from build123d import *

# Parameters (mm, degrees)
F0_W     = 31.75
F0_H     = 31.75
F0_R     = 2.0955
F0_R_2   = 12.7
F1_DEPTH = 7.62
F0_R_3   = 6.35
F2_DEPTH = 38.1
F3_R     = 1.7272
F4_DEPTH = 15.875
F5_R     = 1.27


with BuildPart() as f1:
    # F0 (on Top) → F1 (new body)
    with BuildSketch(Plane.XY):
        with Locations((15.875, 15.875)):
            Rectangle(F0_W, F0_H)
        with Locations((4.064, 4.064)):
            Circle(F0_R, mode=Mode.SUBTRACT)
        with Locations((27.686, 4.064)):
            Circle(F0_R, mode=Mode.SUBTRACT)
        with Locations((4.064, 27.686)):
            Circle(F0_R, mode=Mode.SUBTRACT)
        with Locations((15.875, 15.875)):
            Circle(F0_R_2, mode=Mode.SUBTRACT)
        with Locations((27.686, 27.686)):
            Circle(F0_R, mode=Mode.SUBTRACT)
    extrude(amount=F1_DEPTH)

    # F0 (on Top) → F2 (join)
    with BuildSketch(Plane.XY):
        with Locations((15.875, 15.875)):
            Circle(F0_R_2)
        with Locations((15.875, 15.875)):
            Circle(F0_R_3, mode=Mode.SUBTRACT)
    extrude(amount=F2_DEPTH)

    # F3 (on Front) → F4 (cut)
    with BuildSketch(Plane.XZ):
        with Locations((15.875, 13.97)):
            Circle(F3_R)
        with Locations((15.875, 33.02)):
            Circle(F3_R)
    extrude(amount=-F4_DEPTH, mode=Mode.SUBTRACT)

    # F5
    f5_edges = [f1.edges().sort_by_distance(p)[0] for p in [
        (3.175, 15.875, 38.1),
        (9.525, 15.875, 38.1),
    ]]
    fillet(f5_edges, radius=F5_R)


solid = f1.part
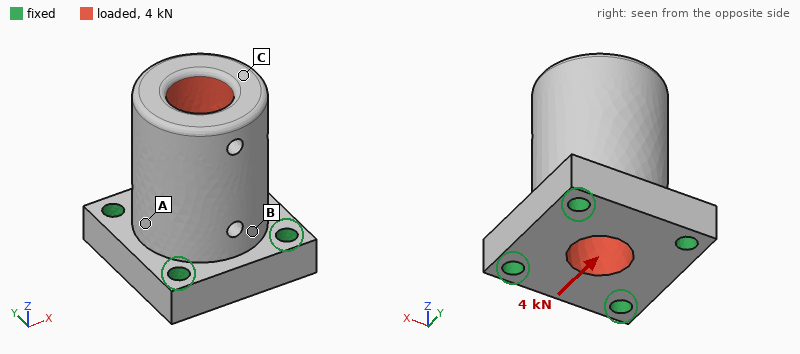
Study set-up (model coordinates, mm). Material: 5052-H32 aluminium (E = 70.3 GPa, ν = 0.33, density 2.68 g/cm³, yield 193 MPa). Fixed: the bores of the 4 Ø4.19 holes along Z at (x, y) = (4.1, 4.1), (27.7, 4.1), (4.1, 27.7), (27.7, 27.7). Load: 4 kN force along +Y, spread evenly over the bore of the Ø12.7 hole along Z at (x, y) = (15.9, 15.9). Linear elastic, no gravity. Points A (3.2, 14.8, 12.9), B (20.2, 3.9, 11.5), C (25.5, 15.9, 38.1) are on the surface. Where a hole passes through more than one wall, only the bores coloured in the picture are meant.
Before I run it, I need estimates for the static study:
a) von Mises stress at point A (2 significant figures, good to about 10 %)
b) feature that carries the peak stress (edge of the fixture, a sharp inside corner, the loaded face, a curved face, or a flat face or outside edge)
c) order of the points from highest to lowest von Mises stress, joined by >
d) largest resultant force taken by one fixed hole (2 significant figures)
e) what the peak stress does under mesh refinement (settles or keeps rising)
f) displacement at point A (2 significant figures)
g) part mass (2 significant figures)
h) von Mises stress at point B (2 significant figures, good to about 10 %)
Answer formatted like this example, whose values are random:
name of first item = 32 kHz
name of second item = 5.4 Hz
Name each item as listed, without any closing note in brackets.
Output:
von Mises stress at point A = 15 MPa
feature that carries the peak stress = edge of the fixture
order of the points from highest to lowest von Mises stress, joined by > = B > A > C
largest resultant force taken by one fixed hole = 1.7 kN
what the peak stress does under mesh refinement = keeps rising
displacement at point A = 6.6 µm
part mass = 47 g
von Mises stress at point B = 25 MPa
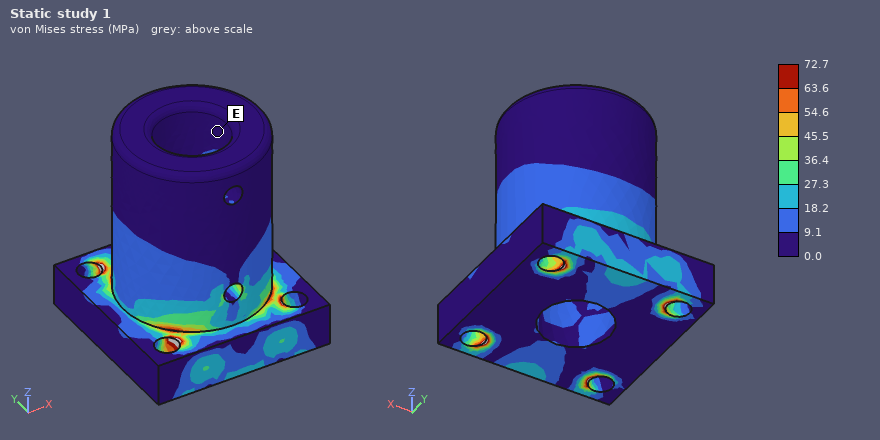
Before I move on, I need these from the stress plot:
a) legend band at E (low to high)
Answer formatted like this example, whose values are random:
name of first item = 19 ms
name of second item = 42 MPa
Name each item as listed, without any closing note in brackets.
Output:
legend band at E = 0.0 to 9.1 MPa
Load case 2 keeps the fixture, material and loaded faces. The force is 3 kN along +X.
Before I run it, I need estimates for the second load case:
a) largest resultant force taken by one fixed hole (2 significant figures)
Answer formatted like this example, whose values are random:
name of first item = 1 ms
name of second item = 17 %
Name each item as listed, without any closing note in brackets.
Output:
largest resultant force taken by one fixed hole = 1.3 kN
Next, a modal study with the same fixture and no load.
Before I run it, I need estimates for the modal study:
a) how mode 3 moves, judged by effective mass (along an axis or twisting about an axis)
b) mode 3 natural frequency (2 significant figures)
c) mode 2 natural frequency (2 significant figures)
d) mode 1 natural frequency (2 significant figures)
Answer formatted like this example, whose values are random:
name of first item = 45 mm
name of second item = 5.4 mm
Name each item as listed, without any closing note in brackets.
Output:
how mode 3 moves, judged by effective mass = twisting about Z
mode 3 natural frequency = 23 kHz
mode 2 natural frequency = 11 kHz
mode 1 natural frequency = 11 kHz
